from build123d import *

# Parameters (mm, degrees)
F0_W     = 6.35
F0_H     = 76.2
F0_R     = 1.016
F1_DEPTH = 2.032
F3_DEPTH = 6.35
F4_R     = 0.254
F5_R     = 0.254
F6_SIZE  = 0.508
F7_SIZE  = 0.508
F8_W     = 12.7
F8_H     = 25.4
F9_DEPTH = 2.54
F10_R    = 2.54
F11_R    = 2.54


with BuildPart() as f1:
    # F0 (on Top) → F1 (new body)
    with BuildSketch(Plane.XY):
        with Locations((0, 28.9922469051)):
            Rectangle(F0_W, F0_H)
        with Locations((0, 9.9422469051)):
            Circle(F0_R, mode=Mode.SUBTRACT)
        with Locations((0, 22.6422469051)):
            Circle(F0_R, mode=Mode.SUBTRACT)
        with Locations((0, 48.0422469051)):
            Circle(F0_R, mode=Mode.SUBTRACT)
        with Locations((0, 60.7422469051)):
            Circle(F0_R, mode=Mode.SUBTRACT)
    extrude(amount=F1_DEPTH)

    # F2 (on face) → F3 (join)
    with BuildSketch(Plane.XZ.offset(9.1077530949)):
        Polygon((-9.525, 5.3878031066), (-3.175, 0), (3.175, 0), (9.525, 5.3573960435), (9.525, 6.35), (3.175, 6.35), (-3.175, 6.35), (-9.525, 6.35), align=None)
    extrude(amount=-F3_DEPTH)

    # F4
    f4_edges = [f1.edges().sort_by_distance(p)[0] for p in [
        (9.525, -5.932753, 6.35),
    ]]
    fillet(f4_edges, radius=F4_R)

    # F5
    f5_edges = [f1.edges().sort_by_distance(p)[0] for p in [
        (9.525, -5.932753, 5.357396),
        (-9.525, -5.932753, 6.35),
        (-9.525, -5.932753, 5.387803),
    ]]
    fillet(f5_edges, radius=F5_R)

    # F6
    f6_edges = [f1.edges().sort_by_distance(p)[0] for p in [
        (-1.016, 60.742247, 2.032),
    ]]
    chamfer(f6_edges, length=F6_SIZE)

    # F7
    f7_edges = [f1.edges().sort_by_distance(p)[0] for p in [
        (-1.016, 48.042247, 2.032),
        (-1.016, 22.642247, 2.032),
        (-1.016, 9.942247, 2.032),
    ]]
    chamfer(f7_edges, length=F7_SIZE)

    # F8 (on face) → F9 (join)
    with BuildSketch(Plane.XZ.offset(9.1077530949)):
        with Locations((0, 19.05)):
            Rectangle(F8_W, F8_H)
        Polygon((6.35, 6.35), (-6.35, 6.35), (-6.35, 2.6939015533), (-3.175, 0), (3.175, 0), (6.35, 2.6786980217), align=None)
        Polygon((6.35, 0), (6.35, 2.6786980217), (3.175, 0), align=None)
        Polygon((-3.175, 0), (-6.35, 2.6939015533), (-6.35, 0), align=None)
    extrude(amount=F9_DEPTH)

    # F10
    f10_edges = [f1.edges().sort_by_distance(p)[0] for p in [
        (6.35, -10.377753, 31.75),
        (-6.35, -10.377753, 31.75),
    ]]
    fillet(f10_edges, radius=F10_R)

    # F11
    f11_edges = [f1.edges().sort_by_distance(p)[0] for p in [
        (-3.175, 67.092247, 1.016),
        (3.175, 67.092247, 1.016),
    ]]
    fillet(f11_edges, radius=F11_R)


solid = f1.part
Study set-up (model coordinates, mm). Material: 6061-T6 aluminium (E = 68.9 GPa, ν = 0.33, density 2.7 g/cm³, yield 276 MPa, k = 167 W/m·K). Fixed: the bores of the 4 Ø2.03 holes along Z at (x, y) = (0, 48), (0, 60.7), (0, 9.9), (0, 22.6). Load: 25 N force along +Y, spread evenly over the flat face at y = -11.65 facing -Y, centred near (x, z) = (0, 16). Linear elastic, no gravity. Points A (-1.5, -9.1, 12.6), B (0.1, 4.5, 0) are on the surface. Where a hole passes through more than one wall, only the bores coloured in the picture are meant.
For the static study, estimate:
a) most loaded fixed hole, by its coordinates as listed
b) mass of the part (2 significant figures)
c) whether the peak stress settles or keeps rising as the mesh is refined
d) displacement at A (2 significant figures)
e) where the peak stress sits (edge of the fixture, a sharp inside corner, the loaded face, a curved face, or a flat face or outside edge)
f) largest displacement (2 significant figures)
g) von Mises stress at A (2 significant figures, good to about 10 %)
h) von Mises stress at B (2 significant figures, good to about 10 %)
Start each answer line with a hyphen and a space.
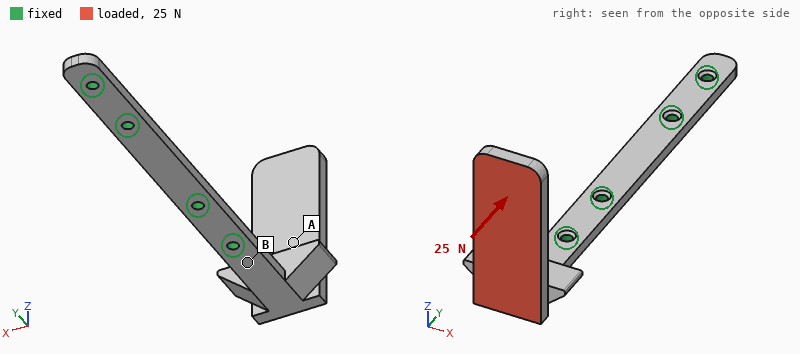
- (0, 9.9)
- 6.6 g
- keeps rising
- 0.28 mm
- edge of the fixture
- 0.60 mm
- 9.8 MPa
- 81 MPa
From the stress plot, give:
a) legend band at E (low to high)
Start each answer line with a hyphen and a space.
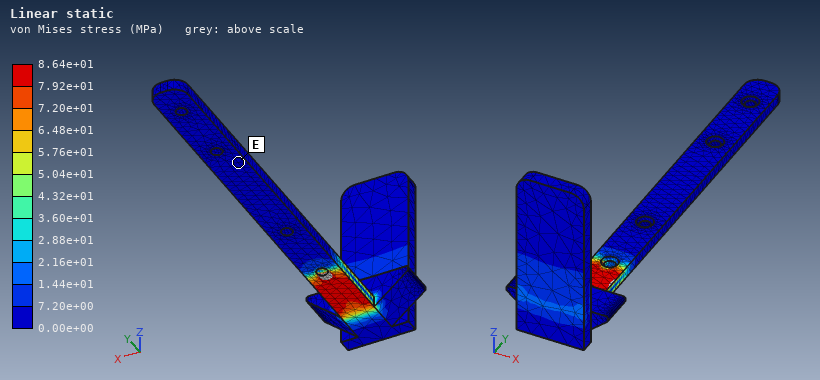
- 0.00e+00 to 7.20e+00 MPa
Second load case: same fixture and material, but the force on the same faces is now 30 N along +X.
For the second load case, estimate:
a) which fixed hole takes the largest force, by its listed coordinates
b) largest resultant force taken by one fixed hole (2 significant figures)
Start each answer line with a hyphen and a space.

- (0, 9.9)
- 56 N
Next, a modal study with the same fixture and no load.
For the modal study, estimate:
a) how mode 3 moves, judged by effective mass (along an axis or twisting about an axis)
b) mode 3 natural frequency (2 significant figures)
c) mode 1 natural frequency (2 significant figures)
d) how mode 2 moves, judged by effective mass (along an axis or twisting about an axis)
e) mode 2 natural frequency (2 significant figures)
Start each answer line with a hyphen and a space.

- along Z
- 2900 Hz
- 610 Hz
- along X
- 880 Hz
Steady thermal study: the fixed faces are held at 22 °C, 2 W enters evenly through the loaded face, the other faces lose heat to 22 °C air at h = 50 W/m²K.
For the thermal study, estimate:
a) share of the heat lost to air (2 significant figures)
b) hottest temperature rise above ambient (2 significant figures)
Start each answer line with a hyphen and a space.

- 28 %
- 14 K
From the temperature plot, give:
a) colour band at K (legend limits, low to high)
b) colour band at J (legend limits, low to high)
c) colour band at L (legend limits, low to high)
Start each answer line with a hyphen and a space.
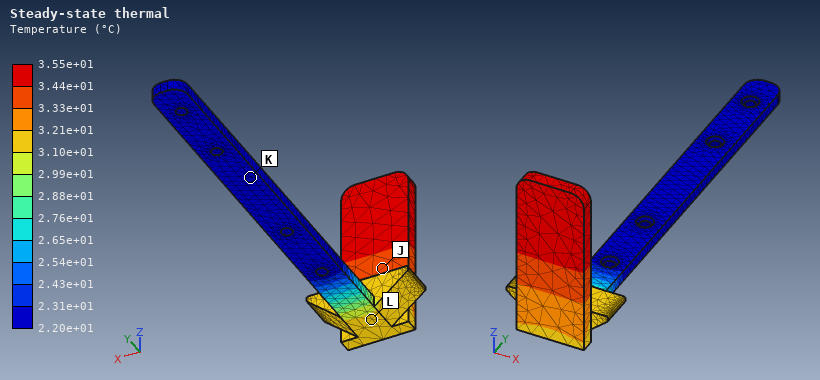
- 2.20e+01 to 2.31e+01 °C
- 3.33e+01 to 3.44e+01 °C
- 3.10e+01 to 3.21e+01 °C
